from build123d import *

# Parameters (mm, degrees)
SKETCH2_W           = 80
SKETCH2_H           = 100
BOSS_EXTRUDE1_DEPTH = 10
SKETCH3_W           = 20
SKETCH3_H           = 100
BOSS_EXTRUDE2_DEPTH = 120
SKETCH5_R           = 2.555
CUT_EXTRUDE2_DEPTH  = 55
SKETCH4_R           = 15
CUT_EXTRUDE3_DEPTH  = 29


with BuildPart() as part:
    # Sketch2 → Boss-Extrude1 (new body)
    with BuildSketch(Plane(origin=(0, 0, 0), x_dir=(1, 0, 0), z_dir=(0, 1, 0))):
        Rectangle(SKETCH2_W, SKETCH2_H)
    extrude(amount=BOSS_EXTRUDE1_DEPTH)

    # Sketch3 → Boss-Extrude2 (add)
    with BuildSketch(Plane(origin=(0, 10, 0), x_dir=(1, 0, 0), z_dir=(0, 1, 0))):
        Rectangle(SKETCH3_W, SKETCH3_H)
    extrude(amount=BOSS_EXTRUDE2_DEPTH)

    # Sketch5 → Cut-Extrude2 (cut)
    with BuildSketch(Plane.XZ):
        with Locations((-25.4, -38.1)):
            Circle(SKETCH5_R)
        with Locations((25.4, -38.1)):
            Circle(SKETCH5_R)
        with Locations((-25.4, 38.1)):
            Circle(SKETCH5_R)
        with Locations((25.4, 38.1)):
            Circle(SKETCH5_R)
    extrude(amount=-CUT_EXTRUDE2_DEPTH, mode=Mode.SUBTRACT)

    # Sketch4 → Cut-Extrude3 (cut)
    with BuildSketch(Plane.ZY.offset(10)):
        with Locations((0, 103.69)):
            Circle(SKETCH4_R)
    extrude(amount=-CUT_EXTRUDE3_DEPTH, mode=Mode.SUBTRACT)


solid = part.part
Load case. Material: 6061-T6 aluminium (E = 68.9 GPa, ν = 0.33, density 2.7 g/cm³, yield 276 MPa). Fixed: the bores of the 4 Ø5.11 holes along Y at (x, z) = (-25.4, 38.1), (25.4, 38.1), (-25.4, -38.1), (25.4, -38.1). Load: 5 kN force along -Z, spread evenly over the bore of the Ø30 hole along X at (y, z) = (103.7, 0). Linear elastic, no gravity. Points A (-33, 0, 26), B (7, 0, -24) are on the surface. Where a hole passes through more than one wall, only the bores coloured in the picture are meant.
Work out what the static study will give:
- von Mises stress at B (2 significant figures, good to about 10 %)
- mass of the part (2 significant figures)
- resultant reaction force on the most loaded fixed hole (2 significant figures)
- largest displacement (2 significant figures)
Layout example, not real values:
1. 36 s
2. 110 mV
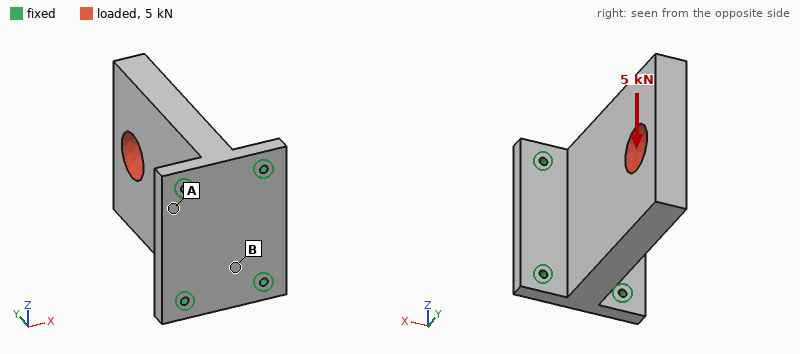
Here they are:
1. 17 MPa
2. 820 g
3. 3.6 kN
4. 0.12 mm
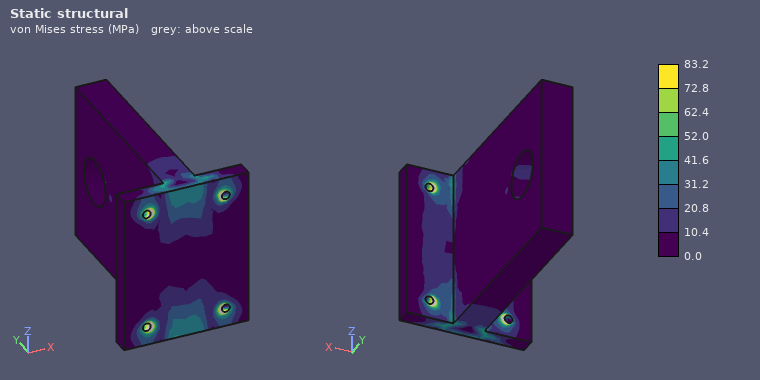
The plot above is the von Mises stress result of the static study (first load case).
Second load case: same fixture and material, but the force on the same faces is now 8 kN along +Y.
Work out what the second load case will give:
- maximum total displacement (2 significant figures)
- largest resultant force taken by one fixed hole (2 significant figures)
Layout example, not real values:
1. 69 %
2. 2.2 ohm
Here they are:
1. 26 µm
2. 2.1 kN
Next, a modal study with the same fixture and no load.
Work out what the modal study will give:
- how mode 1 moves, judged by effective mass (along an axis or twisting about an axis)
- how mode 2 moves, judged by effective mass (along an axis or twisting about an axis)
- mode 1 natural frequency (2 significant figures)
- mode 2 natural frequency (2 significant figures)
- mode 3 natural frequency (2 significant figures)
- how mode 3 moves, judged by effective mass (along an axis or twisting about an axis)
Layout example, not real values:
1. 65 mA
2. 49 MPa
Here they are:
1. along X
2. along Z
3. 880 Hz
4. 2000 Hz
5. 2500 Hz
6. twisting about Y
